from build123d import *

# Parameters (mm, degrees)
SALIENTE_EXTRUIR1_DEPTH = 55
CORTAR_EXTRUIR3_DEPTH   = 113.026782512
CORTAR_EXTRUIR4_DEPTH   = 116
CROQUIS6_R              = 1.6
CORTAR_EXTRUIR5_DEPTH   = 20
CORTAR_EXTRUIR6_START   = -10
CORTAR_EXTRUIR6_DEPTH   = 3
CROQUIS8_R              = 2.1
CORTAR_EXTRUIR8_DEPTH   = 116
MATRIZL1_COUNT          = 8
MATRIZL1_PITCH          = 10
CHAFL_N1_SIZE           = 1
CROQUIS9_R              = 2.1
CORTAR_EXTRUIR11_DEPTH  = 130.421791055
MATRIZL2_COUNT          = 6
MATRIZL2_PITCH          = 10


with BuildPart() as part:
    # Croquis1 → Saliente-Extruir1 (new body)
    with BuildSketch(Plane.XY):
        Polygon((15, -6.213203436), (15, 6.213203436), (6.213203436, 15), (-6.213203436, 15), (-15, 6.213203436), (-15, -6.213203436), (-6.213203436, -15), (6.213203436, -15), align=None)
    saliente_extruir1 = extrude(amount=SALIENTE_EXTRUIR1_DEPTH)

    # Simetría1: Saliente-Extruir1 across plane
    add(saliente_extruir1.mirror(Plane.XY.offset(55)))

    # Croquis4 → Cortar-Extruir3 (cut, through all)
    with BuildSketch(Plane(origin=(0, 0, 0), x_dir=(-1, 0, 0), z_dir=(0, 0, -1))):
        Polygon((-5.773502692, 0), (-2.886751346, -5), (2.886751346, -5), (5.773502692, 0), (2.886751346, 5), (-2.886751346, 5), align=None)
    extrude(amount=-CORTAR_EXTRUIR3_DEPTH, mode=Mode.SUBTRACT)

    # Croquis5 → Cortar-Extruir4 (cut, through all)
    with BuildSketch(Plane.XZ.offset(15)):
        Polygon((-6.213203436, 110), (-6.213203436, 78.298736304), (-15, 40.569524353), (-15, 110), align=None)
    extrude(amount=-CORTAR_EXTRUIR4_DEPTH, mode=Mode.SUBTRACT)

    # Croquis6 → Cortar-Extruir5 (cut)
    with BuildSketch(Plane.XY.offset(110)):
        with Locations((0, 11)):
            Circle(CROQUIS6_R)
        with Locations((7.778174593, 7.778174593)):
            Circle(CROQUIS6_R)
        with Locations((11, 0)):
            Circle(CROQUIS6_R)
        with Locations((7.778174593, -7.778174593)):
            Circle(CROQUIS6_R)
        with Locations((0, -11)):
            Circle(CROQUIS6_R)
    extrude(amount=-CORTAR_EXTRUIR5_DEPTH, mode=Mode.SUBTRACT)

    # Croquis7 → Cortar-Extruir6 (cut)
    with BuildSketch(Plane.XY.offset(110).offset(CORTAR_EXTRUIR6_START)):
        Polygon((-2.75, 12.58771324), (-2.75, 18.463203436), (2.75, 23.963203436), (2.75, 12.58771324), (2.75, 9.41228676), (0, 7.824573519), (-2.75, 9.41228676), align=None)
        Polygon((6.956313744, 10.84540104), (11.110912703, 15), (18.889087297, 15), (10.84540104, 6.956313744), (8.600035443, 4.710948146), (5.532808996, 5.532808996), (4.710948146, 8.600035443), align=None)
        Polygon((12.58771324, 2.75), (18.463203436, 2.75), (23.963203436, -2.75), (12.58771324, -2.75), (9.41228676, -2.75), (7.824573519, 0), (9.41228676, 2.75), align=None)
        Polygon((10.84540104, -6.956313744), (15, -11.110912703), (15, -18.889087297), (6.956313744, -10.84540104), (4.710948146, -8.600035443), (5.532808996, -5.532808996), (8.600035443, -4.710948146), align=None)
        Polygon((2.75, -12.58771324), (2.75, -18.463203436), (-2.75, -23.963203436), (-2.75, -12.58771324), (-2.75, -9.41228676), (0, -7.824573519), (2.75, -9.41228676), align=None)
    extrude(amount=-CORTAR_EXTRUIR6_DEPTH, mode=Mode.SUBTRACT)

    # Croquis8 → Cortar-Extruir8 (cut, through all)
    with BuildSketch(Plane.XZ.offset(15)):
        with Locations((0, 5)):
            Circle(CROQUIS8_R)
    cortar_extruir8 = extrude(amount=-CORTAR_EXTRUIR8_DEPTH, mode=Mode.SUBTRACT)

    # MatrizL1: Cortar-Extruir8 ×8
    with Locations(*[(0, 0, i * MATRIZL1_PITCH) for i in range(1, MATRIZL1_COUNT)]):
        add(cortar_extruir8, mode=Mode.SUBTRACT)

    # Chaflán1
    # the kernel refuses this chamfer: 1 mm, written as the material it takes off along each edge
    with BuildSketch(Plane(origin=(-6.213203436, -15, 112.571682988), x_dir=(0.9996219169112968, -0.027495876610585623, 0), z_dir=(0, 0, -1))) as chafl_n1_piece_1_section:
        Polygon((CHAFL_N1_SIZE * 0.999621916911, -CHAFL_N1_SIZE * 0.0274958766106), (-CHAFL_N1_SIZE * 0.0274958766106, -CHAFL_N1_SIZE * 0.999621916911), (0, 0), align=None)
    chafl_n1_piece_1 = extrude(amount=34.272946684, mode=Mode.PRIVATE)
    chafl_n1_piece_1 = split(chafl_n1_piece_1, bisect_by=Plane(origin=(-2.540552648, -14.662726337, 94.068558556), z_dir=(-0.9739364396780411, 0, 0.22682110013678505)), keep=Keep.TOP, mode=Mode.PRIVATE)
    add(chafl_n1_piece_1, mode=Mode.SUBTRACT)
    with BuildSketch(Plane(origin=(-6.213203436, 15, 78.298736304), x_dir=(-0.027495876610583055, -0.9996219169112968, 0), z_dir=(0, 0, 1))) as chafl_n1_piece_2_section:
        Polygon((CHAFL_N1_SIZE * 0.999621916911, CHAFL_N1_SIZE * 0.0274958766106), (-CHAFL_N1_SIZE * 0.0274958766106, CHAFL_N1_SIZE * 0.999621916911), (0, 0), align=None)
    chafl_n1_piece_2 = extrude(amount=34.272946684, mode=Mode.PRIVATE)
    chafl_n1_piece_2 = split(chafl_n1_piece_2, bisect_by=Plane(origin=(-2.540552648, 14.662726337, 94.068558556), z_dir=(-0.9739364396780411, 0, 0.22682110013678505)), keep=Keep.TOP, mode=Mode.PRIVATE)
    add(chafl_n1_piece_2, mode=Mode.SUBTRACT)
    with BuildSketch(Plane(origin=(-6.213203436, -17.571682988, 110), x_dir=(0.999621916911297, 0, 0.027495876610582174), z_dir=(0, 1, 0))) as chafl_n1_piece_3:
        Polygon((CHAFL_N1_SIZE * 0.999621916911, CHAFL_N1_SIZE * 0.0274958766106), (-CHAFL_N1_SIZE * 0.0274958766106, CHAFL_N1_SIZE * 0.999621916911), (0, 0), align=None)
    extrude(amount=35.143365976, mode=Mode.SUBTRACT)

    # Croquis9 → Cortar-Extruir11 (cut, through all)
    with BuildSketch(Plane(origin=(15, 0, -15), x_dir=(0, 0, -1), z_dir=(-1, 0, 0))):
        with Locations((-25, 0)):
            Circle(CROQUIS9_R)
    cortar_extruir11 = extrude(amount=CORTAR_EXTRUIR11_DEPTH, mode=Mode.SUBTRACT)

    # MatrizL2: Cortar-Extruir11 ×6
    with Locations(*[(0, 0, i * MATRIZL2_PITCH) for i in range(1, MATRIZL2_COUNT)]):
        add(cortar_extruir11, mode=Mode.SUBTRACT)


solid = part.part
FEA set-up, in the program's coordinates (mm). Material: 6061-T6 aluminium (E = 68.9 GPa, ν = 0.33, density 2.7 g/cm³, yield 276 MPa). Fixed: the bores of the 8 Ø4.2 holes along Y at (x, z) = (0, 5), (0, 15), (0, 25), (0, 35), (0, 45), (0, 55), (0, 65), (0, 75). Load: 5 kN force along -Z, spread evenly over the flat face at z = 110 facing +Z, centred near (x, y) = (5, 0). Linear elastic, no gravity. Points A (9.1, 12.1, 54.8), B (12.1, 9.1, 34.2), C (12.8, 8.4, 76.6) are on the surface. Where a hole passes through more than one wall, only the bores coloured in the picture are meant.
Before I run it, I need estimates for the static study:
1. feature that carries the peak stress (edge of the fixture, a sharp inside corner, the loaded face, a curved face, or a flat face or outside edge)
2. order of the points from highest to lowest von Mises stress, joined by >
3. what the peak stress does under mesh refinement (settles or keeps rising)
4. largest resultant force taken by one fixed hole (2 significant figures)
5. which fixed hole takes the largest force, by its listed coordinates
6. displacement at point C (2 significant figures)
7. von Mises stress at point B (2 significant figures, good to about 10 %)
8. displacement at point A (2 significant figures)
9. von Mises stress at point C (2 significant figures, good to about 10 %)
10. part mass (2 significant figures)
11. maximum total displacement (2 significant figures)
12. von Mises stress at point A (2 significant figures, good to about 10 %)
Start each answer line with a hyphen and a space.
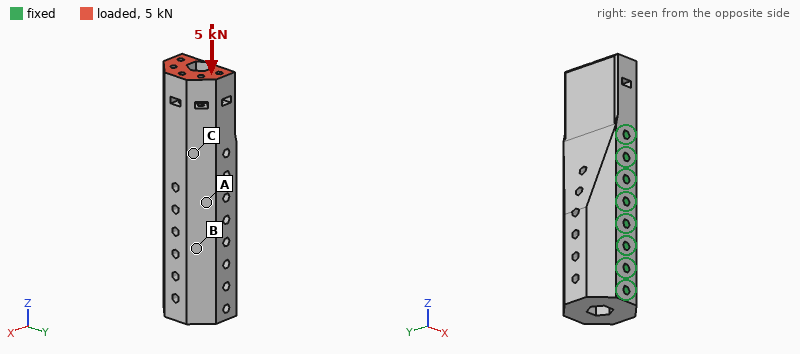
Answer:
- edge of the fixture
- C > A > B
- keeps rising
- 2.2 kN
- (0, 75)
- 7.5 µm
- 3.6 MPa
- 3.6 µm
- 13 MPa
- 160 g
- 20 µm
- 8.2 MPa
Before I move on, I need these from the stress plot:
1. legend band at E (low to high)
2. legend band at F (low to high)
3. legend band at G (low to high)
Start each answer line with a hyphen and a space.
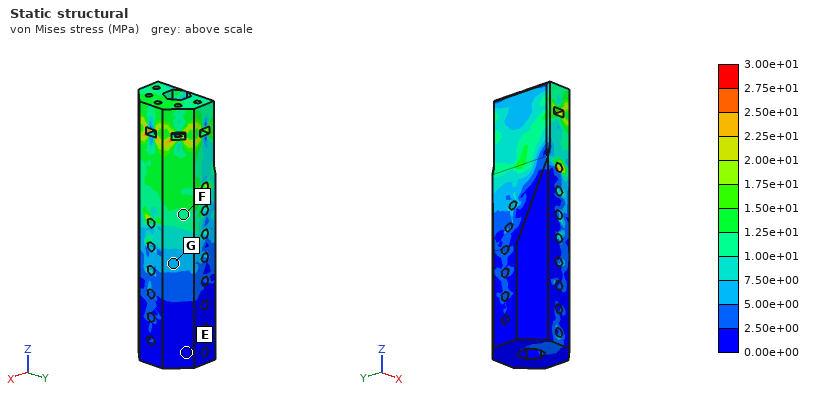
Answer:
- 0.00e+00 to 2.50e+00 MPa
- 1.00e+01 to 1.25e+01 MPa
- 5.00e+00 to 7.50e+00 MPa
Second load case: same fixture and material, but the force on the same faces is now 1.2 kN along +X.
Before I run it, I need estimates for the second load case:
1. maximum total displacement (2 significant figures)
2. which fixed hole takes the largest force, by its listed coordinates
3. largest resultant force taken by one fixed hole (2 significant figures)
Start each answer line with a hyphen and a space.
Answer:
- 47 µm
- (0, 75)
- 2.3 kN
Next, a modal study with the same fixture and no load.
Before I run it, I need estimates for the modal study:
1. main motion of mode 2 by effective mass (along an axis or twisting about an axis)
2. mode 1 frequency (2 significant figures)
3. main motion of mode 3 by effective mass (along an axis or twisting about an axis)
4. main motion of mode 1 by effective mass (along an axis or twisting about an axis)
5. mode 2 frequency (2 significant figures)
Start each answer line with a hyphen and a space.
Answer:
- along Y
- 6900 Hz
- along X
- along X
- 9000 Hz
